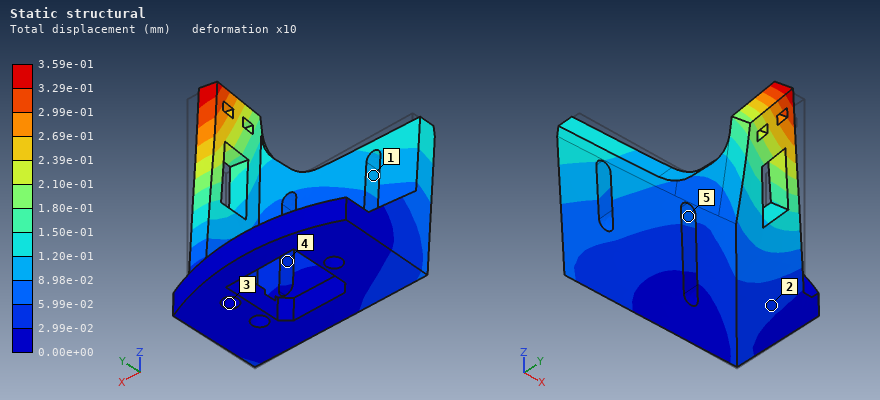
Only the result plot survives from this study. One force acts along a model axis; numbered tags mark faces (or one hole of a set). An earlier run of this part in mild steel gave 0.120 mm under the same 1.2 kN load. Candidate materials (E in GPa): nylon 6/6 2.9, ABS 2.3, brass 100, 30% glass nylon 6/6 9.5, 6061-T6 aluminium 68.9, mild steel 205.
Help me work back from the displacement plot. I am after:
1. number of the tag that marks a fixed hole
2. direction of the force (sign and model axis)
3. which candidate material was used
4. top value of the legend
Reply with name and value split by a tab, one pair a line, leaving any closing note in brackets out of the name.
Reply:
number of the tag that marks a fixed hole	3
direction of the force	-X
which candidate material was used	6061-T6 aluminium
top value of the legend	3.59e-01 mm
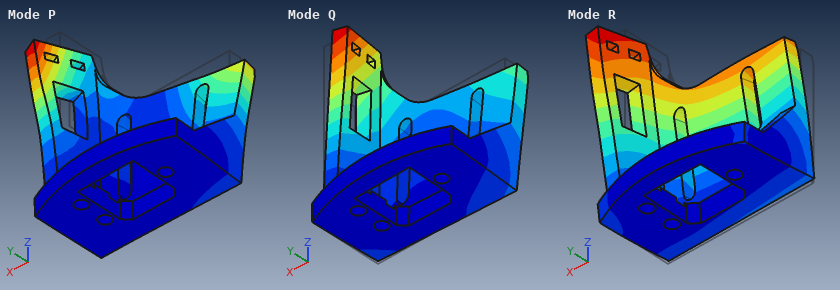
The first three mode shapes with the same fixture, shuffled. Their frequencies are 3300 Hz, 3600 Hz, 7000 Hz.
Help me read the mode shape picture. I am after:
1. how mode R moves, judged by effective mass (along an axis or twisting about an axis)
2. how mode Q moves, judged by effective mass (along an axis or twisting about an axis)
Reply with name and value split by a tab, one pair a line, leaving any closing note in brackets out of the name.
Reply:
how mode R moves, judged by effective mass	along Y
how mode Q moves, judged by effective mass	along X
